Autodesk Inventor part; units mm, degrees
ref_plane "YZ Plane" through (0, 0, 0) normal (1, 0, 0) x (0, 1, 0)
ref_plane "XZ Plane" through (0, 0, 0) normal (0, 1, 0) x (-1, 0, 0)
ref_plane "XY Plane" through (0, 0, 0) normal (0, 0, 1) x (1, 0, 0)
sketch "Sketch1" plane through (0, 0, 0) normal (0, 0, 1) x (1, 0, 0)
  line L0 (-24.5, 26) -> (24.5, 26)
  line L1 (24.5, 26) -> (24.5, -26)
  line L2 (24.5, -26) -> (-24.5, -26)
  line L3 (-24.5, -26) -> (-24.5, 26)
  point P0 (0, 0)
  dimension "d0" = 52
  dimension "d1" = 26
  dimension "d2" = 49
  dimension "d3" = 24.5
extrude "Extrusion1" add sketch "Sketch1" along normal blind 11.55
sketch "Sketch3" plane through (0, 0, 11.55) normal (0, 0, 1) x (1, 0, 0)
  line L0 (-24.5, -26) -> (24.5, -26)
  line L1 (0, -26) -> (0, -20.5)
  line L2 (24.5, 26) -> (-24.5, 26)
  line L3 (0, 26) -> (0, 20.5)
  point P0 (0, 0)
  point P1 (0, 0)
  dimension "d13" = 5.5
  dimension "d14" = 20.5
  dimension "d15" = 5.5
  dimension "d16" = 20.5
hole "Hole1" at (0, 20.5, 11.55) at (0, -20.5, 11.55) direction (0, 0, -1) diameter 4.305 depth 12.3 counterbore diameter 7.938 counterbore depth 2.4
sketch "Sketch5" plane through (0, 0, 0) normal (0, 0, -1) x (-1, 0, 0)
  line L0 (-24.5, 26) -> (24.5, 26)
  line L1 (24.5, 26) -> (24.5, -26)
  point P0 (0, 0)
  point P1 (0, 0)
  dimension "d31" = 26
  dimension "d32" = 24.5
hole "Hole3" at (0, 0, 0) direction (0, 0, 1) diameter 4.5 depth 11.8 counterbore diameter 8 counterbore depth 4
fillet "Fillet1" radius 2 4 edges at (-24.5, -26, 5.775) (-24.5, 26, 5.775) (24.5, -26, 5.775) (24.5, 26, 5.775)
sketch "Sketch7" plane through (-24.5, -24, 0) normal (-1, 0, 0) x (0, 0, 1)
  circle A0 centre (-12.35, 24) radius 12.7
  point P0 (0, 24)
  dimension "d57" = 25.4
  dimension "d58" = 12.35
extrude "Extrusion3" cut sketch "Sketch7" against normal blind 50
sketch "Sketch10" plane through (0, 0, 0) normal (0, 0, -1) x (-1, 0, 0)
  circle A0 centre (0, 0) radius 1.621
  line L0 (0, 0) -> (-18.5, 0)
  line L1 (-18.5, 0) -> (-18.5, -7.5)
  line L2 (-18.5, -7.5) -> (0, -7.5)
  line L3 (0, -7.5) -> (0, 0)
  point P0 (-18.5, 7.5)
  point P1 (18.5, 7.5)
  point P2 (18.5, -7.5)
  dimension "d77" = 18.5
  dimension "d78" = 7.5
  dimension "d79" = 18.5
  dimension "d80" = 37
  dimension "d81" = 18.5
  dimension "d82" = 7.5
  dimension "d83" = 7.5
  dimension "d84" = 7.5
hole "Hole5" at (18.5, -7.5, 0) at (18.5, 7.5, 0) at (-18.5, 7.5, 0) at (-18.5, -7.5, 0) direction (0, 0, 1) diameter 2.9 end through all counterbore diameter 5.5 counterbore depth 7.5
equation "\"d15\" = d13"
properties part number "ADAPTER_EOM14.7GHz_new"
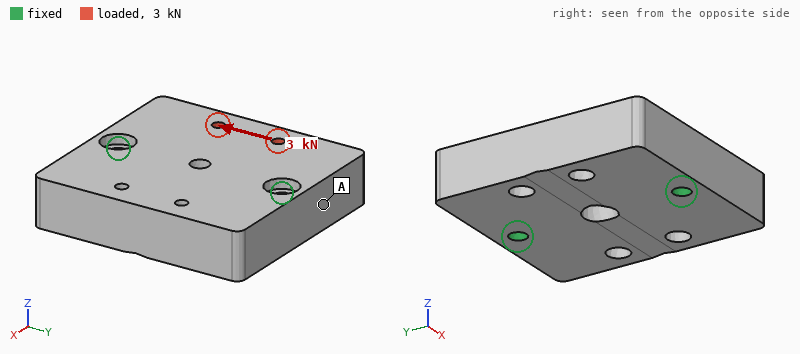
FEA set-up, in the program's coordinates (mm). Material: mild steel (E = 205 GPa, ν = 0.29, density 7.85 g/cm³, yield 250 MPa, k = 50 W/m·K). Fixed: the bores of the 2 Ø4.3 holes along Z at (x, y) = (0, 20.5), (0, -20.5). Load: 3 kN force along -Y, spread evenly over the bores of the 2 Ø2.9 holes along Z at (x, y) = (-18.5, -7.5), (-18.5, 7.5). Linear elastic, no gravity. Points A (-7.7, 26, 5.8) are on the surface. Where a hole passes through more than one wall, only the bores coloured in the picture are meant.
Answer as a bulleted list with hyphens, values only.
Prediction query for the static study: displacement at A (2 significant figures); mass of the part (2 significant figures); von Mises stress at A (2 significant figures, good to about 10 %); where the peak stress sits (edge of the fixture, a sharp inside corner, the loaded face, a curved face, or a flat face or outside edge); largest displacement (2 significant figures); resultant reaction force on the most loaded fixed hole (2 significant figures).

- 1.1 µm
- 220 g
- 6.6 MPa
- the loaded face
- 3.1 µm
- 2.0 kN
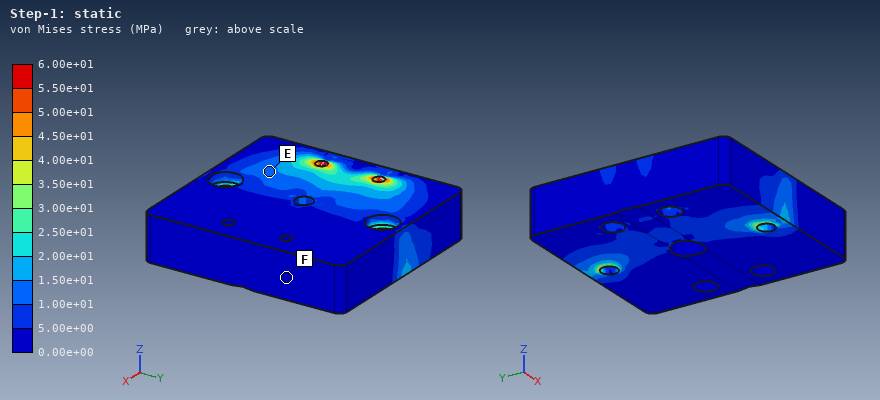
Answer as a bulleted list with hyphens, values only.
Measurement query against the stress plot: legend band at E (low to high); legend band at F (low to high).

- 1.00e+01 to 1.50e+01 MPa
- 0.00e+00 to 5.00e+00 MPa
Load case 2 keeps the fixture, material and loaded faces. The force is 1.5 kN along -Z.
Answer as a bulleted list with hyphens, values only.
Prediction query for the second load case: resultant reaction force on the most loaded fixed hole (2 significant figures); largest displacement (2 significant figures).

- 780 N
- 12 µm
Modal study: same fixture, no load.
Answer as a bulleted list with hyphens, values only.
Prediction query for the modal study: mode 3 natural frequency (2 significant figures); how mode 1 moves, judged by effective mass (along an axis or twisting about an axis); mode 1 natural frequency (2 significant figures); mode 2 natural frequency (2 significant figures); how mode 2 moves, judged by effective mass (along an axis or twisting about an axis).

- 16 kHz
- twisting about Y
- 7800 Hz
- 12 kHz
- along Z
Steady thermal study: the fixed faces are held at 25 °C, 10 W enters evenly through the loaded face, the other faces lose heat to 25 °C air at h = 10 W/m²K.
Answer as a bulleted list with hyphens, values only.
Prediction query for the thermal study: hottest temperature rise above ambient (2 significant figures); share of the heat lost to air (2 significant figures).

- 15 K
- 3.3 %
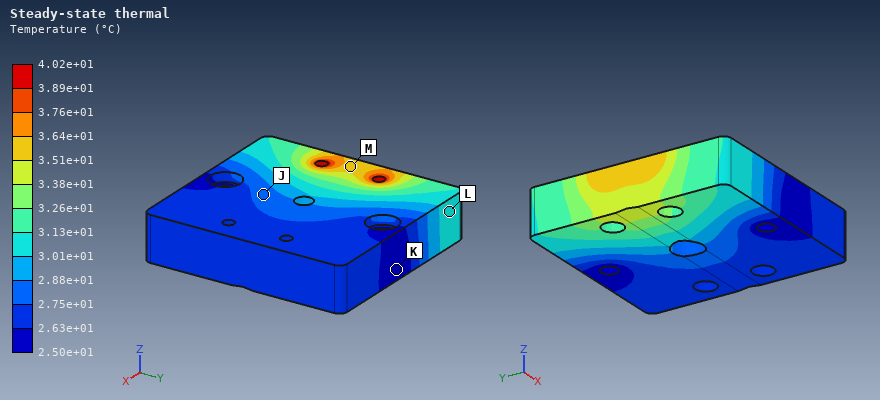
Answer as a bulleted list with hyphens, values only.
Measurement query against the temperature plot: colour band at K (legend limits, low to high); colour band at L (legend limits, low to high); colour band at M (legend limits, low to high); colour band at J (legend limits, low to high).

- 2.50e+01 to 2.63e+01 °C
- 3.01e+01 to 3.13e+01 °C
- 3.51e+01 to 3.64e+01 °C
- 2.75e+01 to 2.88e+01 °C
